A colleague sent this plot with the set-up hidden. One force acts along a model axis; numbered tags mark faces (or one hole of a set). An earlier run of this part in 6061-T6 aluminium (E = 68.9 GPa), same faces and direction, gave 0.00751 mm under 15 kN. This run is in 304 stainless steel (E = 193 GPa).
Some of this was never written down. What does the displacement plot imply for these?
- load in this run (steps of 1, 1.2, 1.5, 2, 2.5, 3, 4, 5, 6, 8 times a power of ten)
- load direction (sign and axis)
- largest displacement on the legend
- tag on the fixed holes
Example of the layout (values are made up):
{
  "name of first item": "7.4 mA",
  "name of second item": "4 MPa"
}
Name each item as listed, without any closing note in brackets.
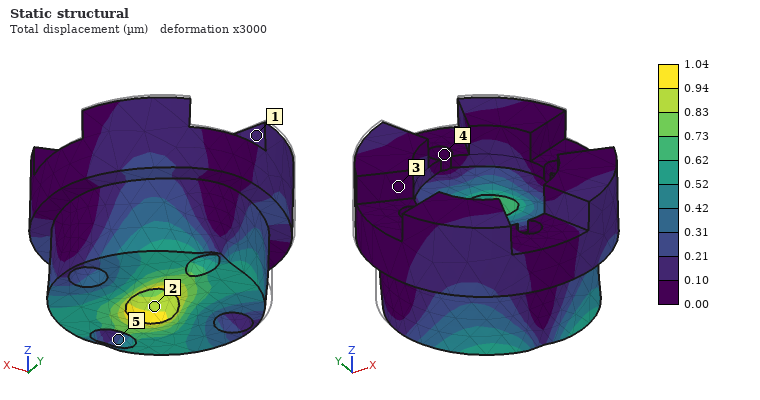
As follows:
{
  "load in this run": "6 kN",
  "load direction": "-Y",
  "largest displacement on the legend": "1.04 µm",
  "tag on the fixed holes": "4"
}
